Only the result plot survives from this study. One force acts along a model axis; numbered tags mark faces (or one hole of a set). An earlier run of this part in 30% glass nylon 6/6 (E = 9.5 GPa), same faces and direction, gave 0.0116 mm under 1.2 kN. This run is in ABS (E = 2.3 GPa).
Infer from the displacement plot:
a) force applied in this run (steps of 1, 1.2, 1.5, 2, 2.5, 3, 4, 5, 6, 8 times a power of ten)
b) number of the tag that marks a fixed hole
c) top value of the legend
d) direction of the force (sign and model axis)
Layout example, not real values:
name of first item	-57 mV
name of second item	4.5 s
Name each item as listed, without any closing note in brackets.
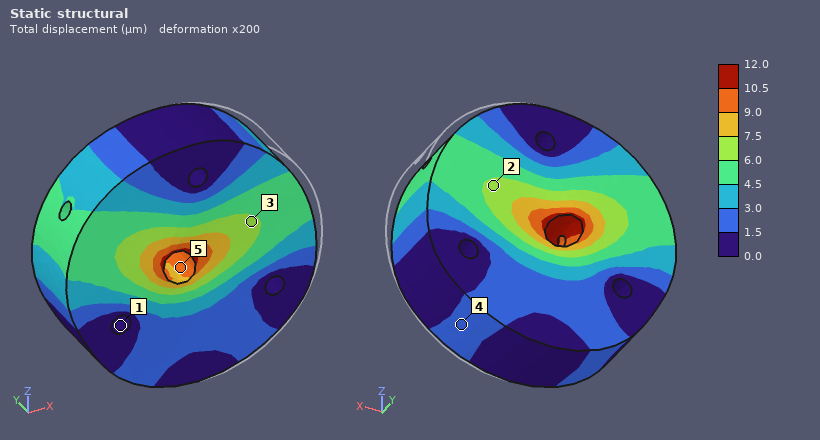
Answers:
force applied in this run	300 N
number of the tag that marks a fixed hole	1
top value of the legend	12.0 µm
direction of the force	-X
